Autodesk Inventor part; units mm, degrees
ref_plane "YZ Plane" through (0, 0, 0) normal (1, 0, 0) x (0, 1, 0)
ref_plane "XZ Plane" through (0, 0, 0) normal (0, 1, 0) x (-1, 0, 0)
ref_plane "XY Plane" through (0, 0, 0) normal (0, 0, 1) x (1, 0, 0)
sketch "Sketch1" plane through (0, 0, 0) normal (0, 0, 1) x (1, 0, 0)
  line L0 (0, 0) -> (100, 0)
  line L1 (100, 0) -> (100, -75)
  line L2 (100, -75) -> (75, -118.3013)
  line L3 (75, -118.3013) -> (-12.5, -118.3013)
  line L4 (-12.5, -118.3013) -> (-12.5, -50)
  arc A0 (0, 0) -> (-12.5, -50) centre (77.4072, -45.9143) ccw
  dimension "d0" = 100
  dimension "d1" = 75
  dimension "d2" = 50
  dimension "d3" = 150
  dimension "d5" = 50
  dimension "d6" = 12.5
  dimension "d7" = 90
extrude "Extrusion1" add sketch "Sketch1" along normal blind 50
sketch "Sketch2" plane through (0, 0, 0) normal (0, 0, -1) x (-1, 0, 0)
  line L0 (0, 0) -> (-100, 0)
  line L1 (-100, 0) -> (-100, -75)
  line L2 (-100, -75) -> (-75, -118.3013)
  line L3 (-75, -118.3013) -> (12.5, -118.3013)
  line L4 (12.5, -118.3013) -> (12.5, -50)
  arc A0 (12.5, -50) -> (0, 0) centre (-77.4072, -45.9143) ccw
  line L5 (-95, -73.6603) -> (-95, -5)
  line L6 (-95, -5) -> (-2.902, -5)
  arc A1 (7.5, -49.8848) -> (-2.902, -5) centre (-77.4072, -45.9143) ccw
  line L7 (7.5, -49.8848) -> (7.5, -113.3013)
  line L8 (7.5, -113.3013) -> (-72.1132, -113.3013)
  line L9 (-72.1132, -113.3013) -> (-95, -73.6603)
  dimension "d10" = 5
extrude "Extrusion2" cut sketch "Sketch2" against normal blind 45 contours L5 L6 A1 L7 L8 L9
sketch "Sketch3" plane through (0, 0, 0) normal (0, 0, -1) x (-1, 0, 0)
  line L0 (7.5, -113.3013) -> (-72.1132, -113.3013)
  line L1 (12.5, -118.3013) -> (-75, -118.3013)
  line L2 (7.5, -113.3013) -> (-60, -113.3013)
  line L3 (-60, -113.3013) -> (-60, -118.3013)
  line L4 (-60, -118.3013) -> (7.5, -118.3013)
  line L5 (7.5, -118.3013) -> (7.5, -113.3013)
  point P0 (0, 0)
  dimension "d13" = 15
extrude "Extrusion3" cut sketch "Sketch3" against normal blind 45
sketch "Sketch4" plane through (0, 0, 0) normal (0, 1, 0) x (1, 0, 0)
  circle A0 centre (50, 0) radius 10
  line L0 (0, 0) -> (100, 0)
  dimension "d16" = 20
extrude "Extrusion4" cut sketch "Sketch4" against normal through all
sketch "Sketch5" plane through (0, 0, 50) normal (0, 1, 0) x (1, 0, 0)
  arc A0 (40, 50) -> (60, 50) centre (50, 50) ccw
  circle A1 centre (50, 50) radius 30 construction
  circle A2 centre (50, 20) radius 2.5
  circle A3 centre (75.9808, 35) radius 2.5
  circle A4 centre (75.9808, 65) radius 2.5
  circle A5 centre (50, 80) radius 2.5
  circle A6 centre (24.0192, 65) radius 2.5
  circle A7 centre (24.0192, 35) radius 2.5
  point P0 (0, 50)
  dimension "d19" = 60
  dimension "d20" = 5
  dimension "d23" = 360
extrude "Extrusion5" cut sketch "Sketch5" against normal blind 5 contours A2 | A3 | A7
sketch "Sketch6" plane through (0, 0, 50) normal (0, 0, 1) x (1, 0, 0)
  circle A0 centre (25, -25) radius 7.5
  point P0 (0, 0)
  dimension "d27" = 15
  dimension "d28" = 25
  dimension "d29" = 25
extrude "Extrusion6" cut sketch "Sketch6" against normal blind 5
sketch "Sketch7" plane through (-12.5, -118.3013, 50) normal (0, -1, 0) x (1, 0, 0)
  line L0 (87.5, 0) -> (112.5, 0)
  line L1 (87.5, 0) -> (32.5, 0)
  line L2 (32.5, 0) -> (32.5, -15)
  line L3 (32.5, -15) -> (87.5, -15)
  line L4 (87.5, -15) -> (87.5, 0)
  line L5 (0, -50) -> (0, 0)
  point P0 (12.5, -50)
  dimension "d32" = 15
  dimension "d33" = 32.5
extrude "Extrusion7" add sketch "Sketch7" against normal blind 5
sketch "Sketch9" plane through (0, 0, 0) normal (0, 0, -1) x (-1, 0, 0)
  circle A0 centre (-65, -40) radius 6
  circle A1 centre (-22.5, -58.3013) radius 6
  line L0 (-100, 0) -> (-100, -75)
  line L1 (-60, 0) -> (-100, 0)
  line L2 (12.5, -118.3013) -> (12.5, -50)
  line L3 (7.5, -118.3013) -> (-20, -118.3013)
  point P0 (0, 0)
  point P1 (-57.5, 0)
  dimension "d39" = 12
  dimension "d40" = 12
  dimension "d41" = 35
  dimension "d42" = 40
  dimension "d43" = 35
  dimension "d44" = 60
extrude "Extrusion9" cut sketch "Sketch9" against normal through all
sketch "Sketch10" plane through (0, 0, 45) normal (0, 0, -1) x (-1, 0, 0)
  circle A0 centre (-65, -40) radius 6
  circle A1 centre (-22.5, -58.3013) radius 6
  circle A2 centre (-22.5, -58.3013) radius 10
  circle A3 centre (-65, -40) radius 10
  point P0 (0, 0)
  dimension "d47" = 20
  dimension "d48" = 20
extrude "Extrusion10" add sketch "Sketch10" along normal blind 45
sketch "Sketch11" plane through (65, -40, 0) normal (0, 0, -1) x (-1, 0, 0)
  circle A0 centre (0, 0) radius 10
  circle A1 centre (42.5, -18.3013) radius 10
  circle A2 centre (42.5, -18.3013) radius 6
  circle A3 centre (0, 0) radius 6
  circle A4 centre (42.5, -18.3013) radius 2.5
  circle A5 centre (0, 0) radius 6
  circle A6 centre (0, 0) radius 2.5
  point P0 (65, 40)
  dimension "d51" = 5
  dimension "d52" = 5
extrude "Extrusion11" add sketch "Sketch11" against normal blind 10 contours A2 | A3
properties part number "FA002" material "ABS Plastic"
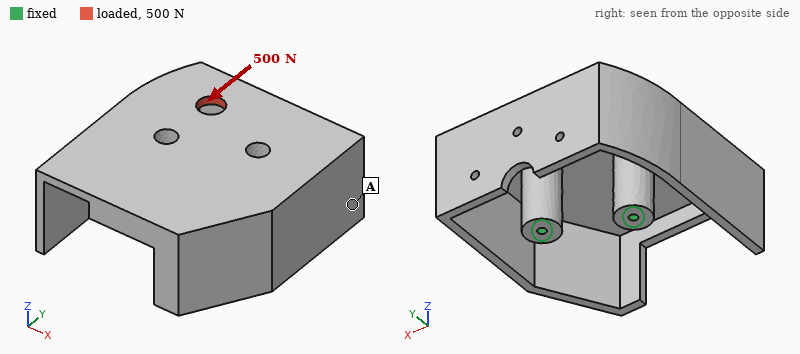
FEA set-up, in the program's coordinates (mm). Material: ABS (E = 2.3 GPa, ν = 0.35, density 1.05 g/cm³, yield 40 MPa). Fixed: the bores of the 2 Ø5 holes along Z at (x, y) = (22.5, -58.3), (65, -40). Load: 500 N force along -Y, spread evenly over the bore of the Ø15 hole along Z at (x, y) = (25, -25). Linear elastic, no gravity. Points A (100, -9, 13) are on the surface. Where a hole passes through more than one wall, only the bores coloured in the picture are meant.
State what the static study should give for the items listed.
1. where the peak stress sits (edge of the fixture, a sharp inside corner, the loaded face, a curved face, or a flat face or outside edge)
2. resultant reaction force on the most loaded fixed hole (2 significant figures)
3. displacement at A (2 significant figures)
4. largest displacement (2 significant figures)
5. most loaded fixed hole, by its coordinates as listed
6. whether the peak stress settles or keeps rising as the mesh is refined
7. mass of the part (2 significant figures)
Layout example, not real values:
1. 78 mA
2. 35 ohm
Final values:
1. edge of the fixture
2. 360 N
3. 0.80 mm
4. 2.0 mm
5. (22.5, -58.3)
6. keeps rising
7. 170 g
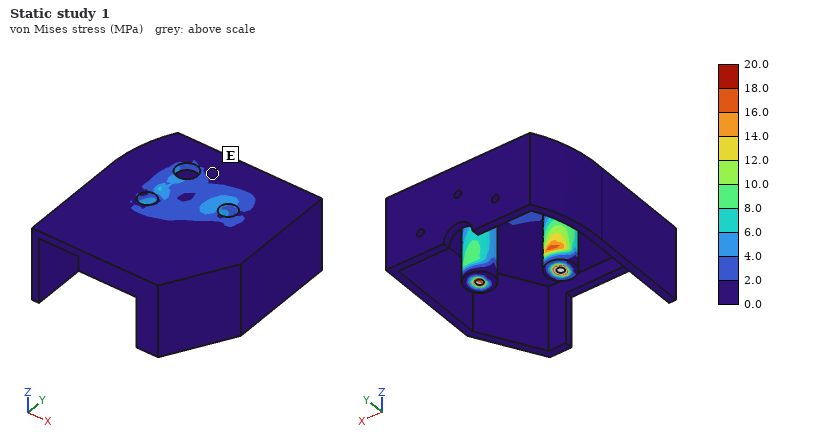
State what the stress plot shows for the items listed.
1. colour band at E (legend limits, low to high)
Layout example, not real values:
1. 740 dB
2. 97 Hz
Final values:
1. 0.0 to 2.0 MPa
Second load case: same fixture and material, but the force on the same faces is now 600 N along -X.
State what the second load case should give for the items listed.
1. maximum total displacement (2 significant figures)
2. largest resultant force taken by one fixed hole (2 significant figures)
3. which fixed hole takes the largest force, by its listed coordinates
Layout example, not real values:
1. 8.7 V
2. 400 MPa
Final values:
1. 1.9 mm
2. 430 N
3. (65, -40)
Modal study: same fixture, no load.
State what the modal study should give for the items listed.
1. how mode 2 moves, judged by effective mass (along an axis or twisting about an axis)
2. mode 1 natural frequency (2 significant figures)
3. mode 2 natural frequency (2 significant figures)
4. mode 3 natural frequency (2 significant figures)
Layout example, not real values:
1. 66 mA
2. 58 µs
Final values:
1. twisting about Z
2. 160 Hz
3. 220 Hz
4. 270 Hz
